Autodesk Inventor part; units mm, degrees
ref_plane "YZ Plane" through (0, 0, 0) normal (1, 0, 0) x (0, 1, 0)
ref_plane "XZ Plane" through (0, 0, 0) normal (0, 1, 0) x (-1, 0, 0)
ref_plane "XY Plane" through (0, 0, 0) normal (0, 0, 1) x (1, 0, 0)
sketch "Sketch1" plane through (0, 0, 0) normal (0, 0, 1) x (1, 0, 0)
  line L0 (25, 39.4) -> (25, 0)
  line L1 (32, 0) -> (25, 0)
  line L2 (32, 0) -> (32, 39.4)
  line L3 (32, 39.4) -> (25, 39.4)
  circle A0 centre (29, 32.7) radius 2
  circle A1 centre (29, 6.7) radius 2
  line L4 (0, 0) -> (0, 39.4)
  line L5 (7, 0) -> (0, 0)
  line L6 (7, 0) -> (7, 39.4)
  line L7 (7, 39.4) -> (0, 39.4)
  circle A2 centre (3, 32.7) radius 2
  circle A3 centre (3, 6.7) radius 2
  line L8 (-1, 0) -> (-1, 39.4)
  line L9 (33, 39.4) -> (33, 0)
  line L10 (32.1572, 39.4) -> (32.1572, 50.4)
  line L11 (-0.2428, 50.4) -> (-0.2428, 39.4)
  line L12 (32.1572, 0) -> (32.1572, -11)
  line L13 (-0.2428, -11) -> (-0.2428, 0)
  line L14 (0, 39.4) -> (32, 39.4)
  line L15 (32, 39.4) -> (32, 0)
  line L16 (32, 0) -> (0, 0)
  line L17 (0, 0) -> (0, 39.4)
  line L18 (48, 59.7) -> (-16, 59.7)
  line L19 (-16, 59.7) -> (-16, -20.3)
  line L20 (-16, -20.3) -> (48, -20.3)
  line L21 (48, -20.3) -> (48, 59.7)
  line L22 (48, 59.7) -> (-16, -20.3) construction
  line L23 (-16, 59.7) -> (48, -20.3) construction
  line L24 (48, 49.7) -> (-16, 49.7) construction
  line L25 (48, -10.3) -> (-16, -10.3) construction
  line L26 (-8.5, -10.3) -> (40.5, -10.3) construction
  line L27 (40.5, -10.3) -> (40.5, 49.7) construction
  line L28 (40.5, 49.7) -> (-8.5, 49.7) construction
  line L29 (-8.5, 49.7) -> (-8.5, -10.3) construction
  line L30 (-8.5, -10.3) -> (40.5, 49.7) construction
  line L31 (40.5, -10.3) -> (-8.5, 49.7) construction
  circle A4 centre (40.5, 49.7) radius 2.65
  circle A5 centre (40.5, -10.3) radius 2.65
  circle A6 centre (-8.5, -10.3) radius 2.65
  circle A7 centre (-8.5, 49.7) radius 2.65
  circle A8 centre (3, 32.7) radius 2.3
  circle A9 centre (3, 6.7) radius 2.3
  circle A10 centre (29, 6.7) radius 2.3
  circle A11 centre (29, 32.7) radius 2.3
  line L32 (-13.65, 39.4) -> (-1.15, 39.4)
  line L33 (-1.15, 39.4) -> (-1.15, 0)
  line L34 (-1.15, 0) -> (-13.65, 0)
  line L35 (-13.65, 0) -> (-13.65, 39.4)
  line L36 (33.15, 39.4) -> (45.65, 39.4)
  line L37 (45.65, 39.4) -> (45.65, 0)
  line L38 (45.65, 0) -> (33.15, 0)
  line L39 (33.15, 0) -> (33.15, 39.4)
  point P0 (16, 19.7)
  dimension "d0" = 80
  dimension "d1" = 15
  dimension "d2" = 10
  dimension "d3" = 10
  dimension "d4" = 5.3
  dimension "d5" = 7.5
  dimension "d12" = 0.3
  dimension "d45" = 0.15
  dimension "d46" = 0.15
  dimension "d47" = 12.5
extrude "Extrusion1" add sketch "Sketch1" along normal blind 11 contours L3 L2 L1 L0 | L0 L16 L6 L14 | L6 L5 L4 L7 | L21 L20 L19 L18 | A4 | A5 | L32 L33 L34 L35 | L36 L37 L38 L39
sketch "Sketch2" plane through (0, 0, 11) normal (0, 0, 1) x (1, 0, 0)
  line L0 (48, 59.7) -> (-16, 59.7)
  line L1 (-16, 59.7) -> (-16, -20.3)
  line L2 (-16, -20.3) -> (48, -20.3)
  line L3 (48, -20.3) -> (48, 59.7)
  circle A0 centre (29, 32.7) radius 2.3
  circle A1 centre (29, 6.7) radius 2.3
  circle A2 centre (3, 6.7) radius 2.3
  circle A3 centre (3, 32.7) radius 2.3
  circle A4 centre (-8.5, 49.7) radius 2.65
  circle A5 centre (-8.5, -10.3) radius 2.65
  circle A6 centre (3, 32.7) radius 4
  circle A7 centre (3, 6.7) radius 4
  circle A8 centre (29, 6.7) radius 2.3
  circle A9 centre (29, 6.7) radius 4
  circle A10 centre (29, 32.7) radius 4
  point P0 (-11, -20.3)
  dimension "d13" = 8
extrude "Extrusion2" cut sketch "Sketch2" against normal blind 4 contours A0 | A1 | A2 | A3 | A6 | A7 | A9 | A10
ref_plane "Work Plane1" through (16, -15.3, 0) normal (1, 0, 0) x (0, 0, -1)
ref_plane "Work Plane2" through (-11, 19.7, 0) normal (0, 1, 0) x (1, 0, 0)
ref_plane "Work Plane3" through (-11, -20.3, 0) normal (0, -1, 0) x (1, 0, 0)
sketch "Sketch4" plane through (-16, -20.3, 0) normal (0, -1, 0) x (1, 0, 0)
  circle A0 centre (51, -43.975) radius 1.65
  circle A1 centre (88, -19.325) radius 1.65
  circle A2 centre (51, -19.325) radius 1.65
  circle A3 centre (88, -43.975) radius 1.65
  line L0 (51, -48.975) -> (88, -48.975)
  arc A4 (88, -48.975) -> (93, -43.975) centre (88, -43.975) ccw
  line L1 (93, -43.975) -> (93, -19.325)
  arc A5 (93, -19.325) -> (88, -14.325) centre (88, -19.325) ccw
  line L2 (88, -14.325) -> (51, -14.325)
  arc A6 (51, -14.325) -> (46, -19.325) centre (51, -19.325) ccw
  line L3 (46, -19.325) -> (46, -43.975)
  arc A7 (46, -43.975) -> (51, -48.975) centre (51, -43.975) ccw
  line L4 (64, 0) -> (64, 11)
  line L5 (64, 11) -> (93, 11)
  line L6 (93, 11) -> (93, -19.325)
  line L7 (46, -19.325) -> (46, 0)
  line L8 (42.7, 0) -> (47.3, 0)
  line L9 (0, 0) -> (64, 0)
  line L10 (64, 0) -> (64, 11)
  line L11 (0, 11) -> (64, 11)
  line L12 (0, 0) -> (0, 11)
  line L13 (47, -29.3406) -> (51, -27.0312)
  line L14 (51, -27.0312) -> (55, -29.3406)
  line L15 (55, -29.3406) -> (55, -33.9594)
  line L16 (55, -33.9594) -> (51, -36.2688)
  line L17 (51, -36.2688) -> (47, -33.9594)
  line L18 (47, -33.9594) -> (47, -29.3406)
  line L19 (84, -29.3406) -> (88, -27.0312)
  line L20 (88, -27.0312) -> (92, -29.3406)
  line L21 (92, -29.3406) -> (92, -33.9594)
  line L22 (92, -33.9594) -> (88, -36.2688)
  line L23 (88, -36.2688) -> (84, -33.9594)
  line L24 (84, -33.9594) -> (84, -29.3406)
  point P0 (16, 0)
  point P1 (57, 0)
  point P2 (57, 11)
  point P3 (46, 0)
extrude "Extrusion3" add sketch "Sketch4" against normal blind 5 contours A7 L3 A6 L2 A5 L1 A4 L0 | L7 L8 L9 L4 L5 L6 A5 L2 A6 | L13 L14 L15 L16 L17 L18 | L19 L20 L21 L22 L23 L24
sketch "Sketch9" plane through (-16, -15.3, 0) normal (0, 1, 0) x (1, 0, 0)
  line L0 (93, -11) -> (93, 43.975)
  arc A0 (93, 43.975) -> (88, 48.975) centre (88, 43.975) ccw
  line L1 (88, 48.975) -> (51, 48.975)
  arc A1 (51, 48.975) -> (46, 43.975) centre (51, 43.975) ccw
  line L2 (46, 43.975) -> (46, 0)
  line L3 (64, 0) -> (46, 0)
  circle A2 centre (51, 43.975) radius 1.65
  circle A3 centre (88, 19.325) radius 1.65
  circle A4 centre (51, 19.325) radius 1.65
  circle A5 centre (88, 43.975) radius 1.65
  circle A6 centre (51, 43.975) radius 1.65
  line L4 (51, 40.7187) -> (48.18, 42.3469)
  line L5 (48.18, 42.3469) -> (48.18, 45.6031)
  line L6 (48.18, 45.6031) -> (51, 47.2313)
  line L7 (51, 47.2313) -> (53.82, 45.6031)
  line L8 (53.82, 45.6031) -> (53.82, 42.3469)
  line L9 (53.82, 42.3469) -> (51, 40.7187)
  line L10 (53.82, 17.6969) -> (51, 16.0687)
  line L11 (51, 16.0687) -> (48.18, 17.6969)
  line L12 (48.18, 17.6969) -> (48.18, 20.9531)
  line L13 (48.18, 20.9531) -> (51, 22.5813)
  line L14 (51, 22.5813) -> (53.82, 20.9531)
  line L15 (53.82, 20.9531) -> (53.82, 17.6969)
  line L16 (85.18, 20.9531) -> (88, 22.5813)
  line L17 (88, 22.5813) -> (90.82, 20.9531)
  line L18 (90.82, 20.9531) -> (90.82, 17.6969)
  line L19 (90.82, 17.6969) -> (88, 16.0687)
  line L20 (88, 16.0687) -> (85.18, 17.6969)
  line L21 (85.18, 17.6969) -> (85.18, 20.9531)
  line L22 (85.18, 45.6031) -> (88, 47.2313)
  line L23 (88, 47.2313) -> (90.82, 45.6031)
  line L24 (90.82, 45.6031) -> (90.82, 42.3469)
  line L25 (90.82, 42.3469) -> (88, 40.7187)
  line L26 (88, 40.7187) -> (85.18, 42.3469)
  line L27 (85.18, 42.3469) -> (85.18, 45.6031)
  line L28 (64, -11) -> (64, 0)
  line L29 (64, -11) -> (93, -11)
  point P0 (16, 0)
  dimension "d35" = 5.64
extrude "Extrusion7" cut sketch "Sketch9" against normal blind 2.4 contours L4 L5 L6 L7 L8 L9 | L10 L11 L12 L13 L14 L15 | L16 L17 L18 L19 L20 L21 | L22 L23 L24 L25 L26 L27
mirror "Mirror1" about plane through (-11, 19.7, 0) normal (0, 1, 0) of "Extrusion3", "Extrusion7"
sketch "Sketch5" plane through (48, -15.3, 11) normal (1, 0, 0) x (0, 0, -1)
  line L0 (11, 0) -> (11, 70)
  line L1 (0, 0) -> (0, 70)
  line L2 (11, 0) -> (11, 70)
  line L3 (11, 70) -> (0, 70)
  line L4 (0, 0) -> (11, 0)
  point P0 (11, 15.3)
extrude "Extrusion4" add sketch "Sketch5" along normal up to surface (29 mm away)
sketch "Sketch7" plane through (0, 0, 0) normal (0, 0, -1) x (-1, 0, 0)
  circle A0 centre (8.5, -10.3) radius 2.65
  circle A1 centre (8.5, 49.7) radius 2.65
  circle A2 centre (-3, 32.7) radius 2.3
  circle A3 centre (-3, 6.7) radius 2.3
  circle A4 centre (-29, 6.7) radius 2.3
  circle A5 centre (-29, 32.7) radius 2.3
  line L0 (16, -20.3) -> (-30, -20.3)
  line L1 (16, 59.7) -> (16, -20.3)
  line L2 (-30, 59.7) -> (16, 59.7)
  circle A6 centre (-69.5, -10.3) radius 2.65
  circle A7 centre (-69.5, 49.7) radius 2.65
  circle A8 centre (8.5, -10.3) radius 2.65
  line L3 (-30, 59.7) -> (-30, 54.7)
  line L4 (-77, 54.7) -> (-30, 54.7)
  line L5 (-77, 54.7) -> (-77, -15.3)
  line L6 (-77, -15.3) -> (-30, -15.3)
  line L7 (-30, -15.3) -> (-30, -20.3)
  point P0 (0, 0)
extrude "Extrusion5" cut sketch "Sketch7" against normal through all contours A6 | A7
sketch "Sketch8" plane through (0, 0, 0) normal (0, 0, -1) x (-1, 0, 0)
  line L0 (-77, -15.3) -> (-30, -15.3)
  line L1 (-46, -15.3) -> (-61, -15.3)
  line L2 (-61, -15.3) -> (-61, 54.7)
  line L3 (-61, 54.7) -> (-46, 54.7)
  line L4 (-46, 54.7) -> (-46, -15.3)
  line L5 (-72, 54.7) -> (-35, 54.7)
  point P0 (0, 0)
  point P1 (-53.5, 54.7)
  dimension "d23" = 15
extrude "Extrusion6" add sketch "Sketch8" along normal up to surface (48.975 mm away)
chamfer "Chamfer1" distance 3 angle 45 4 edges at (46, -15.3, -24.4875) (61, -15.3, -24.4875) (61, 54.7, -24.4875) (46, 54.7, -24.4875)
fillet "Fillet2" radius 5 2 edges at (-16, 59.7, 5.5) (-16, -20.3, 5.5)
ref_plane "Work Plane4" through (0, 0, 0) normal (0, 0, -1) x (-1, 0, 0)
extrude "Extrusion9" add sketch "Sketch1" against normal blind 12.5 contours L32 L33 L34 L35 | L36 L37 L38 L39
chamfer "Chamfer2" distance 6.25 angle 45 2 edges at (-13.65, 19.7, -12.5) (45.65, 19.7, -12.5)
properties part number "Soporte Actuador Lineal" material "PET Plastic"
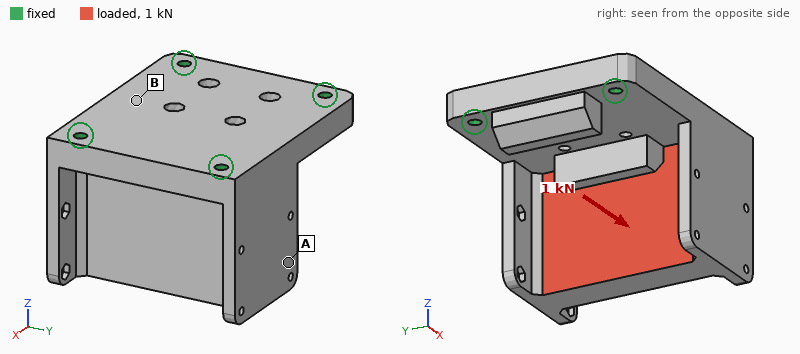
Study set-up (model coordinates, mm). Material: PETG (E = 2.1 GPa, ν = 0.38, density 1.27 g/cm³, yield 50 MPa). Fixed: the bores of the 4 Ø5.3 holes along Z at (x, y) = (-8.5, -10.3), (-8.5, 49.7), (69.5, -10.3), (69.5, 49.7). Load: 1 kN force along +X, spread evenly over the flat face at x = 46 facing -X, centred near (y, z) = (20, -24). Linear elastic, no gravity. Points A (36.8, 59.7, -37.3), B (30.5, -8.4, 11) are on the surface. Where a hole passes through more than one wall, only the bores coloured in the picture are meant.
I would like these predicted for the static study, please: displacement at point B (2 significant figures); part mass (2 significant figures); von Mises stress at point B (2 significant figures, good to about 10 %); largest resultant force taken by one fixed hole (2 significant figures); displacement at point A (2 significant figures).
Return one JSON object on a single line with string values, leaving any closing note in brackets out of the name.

{"displacement at point B": "0.16 mm", "part mass": "210 g", "von Mises stress at point B": "4.6 MPa", "largest resultant force taken by one fixed hole": "380 N", "displacement at point A": "0.38 mm"}
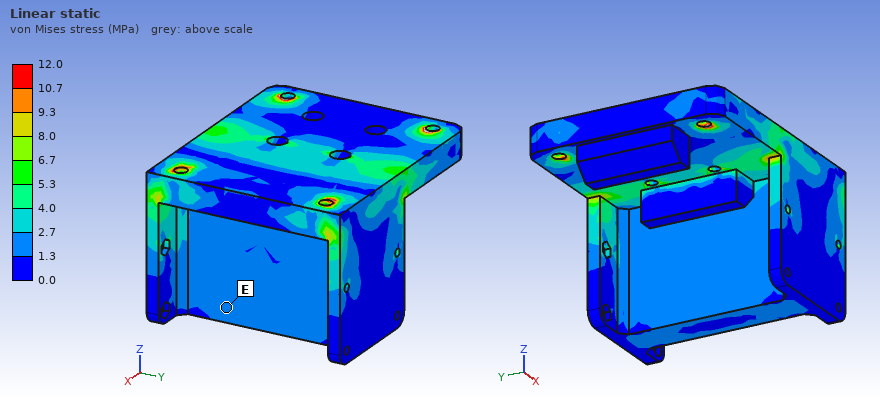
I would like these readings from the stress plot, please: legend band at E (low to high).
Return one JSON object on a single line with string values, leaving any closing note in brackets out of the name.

{"legend band at E": "1.3 to 2.7 MPa"}
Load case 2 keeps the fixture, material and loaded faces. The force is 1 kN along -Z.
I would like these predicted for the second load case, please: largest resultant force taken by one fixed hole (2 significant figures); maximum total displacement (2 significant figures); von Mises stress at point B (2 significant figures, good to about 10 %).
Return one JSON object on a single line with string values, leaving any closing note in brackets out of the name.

{"largest resultant force taken by one fixed hole": "370 N", "maximum total displacement": "0.33 mm", "von Mises stress at point B": "3.4 MPa"}
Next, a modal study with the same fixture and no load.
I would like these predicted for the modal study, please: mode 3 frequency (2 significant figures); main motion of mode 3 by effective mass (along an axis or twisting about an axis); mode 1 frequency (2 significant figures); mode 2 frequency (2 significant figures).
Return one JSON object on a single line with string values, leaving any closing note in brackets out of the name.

{"mode 3 frequency": "1800 Hz", "main motion of mode 3 by effective mass": "along Y", "mode 1 frequency": "810 Hz", "mode 2 frequency": "1200 Hz"}
